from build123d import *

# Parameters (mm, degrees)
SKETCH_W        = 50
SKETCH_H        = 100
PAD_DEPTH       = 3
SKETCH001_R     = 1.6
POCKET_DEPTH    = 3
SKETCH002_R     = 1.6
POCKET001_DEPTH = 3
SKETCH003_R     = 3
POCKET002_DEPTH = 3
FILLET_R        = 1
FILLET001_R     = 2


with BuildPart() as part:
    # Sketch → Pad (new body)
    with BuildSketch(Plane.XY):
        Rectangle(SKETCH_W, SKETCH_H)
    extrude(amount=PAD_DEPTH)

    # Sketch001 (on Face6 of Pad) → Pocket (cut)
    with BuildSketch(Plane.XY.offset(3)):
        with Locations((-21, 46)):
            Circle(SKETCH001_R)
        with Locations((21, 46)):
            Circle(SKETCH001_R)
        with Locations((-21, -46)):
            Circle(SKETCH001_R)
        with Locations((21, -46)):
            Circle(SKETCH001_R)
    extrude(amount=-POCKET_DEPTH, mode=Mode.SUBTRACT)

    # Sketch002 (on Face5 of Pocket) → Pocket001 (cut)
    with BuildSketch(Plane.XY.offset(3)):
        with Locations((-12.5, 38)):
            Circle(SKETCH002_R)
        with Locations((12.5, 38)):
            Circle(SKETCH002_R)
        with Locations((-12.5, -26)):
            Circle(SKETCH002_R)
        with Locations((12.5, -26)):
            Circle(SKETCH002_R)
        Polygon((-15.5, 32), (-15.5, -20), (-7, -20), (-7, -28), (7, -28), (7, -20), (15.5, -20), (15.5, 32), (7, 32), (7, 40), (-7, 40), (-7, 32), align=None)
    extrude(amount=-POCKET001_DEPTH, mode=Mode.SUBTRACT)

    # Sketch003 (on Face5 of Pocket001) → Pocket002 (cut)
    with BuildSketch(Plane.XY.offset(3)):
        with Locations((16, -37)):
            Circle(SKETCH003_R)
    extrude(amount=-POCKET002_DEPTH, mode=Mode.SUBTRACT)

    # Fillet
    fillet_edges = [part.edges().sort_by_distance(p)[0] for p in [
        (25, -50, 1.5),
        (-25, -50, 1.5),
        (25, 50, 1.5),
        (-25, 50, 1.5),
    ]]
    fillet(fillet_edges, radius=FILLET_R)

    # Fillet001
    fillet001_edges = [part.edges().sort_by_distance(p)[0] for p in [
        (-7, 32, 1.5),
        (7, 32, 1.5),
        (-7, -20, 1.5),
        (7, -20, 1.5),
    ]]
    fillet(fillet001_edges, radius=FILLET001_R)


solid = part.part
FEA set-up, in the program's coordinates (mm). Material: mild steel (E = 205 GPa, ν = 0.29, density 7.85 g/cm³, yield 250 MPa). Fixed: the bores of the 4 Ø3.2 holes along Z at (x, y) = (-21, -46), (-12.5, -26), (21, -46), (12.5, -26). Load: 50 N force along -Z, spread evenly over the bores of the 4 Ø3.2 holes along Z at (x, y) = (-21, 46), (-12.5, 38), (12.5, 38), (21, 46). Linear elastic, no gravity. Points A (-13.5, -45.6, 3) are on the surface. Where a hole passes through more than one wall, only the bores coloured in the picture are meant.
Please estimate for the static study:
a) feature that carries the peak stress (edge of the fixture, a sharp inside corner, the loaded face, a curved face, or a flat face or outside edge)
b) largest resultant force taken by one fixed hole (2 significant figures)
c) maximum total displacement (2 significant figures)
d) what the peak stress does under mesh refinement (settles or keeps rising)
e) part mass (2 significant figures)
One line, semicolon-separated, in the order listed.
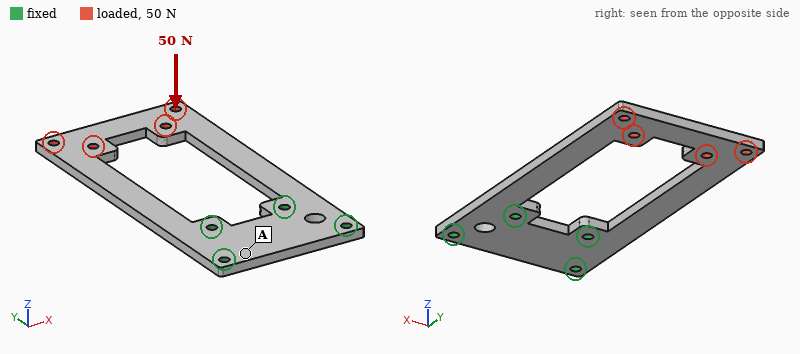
edge of the fixture; 63 N; 0.70 mm; keeps rising; 72 g
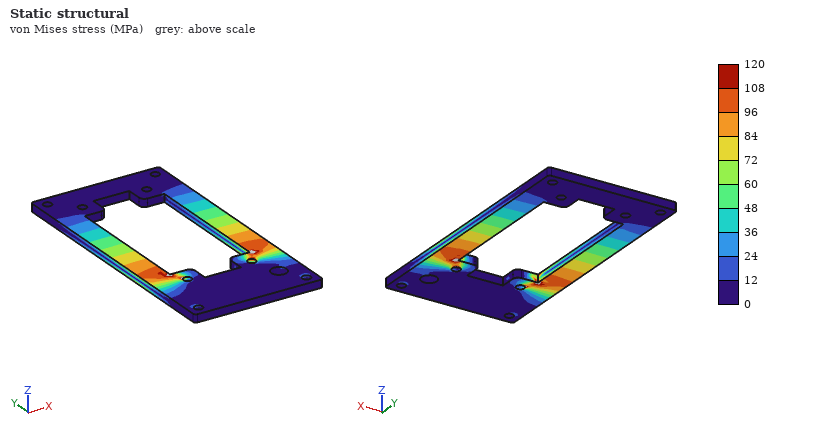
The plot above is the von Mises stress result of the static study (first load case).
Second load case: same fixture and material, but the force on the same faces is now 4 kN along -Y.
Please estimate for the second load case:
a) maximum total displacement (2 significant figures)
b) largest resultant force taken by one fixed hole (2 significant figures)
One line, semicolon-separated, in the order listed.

41 µm; 1.3 kN
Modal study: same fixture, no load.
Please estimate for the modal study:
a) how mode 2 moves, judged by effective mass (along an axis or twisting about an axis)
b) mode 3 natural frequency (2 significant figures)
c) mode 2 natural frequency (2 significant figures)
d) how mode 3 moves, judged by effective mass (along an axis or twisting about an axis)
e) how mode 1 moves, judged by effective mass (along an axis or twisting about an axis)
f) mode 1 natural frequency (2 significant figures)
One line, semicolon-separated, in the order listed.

twisting about Y; 1800 Hz; 960 Hz; along X; along Z; 310 Hz
